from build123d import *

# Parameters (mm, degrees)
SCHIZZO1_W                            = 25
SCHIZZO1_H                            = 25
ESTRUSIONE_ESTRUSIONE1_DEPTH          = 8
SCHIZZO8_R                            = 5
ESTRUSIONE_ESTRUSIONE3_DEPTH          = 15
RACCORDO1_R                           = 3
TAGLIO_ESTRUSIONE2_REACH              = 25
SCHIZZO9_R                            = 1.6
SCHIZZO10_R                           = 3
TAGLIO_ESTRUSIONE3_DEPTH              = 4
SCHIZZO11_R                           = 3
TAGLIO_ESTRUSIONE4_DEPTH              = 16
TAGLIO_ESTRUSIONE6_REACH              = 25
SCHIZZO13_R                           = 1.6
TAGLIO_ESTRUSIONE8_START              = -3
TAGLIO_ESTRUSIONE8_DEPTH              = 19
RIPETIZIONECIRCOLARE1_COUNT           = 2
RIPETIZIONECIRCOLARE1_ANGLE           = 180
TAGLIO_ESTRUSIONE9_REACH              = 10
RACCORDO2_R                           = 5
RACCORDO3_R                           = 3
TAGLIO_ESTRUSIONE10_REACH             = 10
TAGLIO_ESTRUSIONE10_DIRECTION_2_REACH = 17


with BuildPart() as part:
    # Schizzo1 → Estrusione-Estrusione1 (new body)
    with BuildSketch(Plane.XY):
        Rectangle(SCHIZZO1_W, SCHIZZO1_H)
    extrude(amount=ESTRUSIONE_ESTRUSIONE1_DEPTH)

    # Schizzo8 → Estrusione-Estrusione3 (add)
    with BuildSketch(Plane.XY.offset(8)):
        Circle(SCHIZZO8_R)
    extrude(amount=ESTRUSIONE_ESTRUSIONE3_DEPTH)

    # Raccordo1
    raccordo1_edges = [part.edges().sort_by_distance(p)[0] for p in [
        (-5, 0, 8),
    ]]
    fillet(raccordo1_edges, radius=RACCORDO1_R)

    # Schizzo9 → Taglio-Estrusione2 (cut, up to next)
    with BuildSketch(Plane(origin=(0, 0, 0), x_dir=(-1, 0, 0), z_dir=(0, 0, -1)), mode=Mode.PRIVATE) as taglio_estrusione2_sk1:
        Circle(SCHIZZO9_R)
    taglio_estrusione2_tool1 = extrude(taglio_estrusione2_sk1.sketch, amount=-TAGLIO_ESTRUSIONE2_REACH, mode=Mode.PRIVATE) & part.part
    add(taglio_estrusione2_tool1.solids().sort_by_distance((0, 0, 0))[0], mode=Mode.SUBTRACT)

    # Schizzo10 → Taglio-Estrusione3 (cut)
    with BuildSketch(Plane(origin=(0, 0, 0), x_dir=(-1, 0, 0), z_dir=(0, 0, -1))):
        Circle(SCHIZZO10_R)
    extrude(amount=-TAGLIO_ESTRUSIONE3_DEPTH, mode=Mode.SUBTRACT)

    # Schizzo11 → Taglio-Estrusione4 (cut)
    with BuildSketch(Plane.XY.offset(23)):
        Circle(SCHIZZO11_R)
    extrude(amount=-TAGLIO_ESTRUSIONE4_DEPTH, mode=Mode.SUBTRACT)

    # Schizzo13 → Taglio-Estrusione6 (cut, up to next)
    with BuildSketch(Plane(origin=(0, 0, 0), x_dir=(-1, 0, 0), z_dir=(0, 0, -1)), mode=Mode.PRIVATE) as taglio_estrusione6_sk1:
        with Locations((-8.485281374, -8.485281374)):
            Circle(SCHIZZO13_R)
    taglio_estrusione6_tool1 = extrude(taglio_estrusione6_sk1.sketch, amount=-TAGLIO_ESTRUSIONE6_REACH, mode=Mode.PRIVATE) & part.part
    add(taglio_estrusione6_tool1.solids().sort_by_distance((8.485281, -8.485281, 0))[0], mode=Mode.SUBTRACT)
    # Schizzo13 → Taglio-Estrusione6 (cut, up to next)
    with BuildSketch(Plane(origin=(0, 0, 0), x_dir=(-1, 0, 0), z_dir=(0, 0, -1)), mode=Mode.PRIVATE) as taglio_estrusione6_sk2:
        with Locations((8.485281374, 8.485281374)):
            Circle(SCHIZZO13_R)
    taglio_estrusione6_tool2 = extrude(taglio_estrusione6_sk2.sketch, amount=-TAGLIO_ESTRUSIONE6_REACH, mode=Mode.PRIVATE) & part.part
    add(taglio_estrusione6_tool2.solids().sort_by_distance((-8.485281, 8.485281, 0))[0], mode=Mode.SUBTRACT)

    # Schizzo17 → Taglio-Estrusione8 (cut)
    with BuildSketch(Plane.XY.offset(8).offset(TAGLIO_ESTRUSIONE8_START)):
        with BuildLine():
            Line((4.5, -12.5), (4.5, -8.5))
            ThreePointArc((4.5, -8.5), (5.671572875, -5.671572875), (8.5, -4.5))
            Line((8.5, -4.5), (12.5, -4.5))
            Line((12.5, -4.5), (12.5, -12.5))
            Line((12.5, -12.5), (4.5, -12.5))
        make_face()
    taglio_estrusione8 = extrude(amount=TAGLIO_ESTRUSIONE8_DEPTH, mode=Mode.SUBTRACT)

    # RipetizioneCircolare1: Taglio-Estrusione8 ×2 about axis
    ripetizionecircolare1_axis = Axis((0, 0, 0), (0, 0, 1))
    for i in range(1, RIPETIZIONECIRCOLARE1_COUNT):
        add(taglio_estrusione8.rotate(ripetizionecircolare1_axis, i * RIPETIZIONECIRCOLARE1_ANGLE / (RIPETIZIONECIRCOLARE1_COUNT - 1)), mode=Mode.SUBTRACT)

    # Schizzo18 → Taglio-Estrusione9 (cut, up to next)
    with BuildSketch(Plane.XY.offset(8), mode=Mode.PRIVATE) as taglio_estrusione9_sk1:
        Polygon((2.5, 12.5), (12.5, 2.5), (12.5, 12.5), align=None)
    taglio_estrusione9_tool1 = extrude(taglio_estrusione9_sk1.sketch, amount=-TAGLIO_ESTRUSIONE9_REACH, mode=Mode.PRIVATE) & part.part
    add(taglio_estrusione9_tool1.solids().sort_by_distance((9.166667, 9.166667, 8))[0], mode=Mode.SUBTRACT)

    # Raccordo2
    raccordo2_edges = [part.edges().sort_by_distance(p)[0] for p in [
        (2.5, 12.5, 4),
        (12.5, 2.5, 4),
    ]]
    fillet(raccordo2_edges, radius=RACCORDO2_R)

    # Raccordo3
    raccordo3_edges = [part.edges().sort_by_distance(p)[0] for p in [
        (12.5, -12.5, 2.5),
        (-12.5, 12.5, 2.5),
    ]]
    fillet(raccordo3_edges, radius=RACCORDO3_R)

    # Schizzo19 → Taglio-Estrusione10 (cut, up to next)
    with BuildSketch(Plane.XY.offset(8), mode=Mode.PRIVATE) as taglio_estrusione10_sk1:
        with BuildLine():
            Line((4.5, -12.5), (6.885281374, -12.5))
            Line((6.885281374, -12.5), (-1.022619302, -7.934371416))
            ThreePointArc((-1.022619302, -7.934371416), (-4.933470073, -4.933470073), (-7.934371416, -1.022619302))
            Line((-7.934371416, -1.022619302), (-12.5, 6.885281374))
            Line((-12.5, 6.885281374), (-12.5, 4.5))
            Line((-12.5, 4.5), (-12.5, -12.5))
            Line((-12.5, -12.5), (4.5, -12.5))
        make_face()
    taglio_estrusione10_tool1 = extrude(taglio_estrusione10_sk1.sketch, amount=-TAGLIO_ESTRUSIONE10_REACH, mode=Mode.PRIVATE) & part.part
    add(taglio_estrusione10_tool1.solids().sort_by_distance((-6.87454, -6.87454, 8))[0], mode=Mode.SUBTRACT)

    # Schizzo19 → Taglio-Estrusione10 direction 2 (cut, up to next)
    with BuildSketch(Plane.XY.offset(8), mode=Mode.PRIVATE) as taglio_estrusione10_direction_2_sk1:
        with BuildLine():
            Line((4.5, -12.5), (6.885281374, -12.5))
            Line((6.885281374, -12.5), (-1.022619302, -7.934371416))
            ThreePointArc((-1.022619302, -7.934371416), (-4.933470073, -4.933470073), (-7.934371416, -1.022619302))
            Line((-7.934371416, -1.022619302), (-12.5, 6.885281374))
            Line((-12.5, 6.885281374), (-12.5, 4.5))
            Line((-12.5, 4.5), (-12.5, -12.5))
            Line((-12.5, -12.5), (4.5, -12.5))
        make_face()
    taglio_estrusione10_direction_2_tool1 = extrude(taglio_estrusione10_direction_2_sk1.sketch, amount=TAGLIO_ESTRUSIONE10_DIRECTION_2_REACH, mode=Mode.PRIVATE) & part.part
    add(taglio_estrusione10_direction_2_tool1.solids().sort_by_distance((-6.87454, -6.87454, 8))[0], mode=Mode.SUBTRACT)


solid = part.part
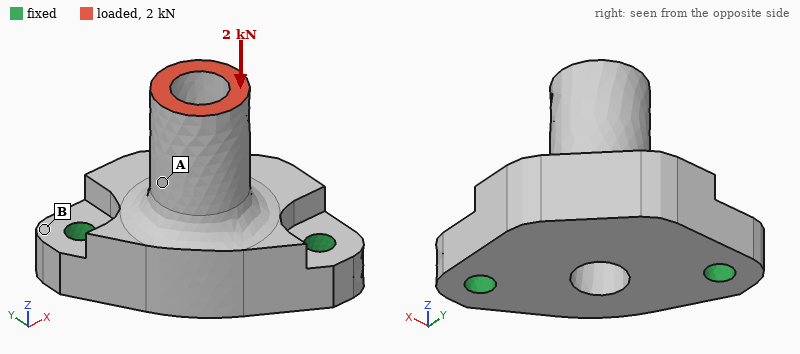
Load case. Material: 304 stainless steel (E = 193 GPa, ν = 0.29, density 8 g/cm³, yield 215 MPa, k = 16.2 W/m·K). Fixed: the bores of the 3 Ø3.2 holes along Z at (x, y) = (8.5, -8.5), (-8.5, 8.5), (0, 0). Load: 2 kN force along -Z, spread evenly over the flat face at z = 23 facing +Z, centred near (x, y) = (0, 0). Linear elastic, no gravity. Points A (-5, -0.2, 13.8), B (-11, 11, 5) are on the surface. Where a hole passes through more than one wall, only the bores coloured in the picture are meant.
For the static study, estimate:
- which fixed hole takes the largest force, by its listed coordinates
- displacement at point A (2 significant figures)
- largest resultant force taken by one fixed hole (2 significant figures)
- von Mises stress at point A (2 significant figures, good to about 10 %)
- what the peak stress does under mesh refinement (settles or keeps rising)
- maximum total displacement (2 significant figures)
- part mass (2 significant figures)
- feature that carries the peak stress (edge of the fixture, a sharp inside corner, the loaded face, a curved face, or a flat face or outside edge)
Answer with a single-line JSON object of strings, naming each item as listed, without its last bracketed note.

{"which fixed hole takes the largest force, by its listed coordinates": "(0, 0)", "displacement at point A": "2.2 µm", "largest resultant force taken by one fixed hole": "1.2 kN", "von Mises stress at point A": "38 MPa", "what the peak stress does under mesh refinement": "keeps rising", "maximum total displacement": "4.1 µm", "part mass": "29 g", "feature that carries the peak stress": "edge of the fixture"}
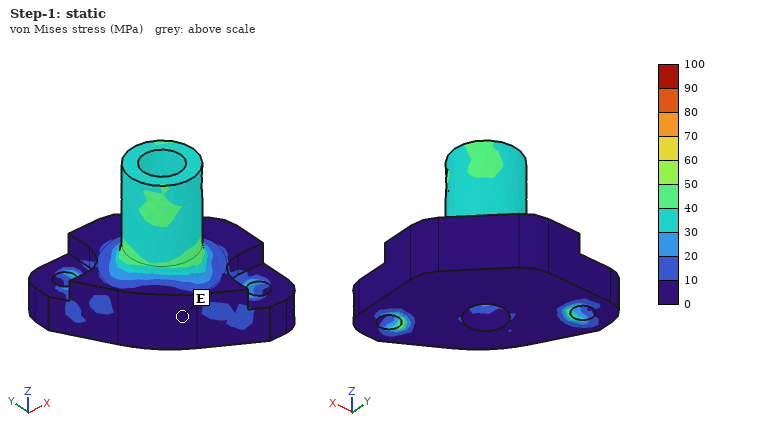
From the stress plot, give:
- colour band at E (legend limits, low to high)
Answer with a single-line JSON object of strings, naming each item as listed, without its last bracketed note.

{"colour band at E": "0 to 10 MPa"}
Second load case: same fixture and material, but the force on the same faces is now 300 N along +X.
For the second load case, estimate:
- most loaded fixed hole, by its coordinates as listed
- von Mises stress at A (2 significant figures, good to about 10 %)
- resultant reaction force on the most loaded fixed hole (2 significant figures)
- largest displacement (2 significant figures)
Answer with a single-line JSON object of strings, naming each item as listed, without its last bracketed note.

{"most loaded fixed hole, by its coordinates as listed": "(0, 0)", "von Mises stress at A": "31 MPa", "resultant reaction force on the most loaded fixed hole": "460 N", "largest displacement": "9.4 µm"}
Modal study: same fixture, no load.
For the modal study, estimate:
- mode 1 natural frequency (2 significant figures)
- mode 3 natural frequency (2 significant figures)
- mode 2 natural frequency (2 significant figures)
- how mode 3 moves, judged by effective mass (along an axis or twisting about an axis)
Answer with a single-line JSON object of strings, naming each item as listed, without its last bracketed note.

{"mode 1 natural frequency": "17 kHz", "mode 3 natural frequency": "38 kHz", "mode 2 natural frequency": "24 kHz", "how mode 3 moves, judged by effective mass": "along Z"}
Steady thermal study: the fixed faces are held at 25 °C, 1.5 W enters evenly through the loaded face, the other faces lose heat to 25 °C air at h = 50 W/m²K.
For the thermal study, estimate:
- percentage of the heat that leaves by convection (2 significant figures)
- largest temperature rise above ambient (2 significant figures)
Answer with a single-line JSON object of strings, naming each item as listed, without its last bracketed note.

{"percentage of the heat that leaves by convection": "35 %", "largest temperature rise above ambient": "24 K"}
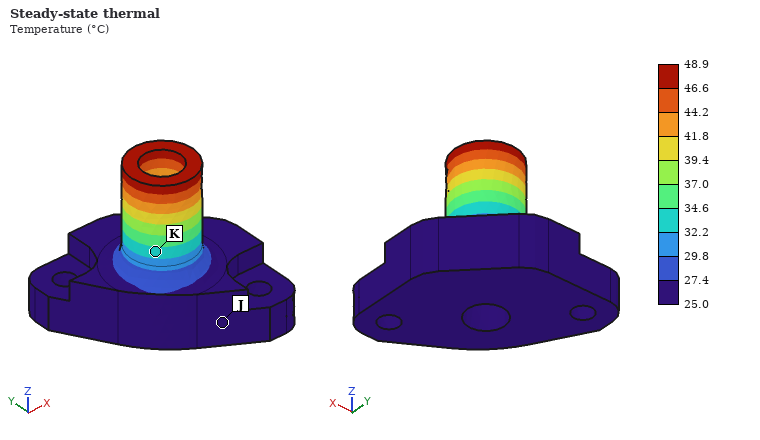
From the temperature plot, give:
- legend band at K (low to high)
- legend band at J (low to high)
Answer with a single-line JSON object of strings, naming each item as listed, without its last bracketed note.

{"legend band at K": "32.2 to 34.6 °C", "legend band at J": "25.0 to 27.4 °C"}
